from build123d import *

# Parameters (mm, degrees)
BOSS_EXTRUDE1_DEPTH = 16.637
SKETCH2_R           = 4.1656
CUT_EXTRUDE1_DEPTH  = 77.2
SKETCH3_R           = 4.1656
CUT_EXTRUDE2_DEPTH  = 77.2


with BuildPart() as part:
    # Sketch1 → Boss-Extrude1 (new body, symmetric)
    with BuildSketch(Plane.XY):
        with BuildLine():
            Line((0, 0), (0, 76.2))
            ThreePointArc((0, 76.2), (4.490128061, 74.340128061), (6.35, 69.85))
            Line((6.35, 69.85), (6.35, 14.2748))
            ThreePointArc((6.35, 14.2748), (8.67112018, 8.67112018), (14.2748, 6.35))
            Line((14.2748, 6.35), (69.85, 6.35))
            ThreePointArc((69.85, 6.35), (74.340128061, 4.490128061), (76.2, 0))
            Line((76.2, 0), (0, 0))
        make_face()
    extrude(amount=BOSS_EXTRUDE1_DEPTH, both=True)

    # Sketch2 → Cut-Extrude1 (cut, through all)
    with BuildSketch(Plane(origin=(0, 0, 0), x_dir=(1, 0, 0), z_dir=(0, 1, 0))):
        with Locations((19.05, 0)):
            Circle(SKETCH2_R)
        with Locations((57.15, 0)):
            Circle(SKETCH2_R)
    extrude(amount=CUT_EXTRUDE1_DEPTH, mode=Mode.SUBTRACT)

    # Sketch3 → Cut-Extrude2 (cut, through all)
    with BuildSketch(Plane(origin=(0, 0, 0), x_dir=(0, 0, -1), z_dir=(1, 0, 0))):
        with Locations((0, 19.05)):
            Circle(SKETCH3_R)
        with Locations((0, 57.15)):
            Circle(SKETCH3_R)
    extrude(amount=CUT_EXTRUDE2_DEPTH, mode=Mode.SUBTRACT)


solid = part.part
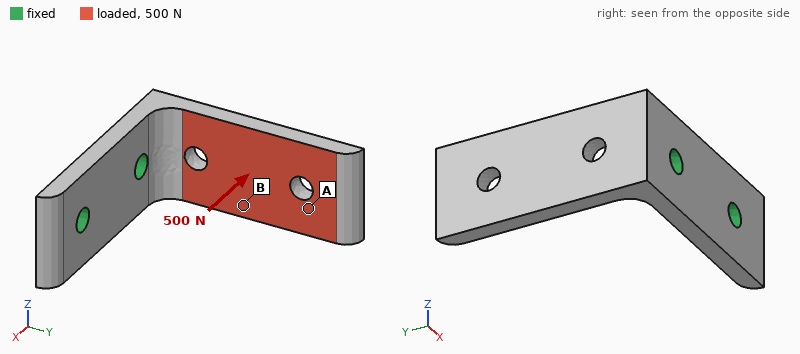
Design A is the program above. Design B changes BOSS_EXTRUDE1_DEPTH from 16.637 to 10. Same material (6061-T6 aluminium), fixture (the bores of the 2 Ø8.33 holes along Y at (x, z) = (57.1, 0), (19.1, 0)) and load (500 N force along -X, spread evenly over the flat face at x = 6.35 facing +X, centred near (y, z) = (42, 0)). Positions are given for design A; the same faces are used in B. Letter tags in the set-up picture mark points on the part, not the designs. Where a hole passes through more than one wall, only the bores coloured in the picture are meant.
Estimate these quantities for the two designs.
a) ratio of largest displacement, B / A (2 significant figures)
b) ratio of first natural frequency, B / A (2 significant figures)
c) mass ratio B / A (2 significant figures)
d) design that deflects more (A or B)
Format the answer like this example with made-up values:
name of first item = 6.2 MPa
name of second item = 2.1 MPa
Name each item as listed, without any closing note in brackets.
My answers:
ratio of largest displacement, B / A = 1.7
ratio of first natural frequency, B / A = 1.0
mass ratio B / A = 0.58
design that deflects more = B
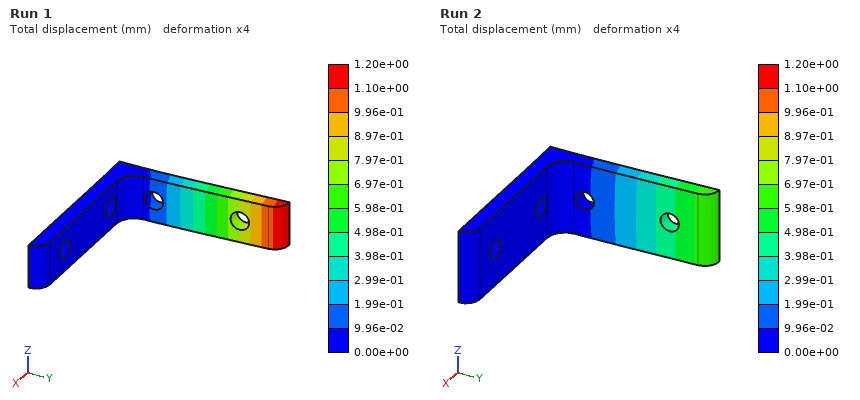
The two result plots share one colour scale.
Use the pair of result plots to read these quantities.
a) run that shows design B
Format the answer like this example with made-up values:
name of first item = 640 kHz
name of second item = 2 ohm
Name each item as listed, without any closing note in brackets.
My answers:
run that shows design B = Run 1
